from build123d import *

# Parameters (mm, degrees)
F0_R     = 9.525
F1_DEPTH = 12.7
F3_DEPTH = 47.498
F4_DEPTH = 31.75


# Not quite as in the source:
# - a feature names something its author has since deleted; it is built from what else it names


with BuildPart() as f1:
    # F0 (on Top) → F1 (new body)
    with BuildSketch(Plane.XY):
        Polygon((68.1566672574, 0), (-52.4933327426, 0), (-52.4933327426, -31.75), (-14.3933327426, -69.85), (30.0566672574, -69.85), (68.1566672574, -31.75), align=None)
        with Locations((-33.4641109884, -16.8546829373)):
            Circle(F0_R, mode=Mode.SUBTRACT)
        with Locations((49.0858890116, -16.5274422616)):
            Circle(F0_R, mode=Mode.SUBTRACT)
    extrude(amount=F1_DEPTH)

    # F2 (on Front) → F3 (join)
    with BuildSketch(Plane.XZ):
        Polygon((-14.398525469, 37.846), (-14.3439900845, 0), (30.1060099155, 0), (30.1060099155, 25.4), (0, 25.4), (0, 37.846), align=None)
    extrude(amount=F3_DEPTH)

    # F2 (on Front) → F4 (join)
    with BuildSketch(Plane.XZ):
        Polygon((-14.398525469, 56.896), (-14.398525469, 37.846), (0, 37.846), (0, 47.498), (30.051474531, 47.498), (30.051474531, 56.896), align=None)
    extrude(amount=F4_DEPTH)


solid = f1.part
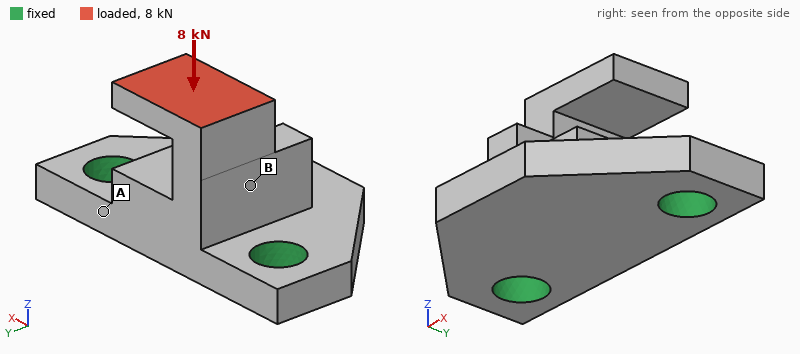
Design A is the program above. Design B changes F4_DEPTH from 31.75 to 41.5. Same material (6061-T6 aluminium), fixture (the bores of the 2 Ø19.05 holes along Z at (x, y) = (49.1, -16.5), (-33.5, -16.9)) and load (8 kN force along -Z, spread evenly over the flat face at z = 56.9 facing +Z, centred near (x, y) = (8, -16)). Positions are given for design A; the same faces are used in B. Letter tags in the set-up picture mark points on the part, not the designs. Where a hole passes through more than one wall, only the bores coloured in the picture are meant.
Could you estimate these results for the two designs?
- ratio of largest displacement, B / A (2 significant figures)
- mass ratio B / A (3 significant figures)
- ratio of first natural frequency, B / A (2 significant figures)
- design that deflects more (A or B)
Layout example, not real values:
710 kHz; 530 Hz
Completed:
0.78; 1.04; 0.94; A
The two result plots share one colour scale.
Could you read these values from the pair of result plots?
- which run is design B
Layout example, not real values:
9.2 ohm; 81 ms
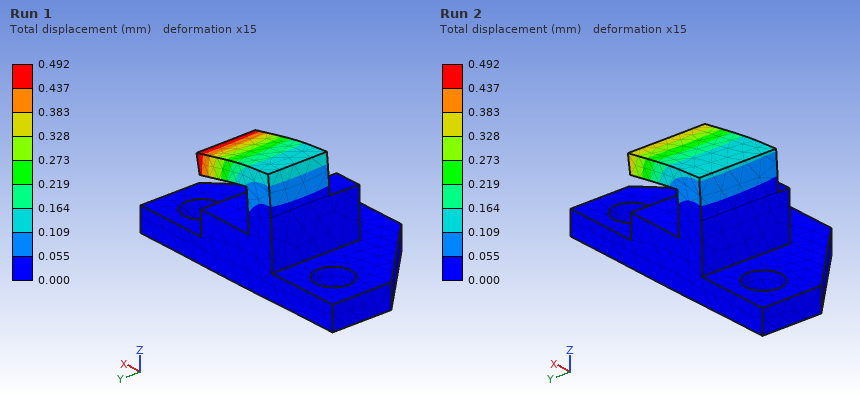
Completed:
Run 2
